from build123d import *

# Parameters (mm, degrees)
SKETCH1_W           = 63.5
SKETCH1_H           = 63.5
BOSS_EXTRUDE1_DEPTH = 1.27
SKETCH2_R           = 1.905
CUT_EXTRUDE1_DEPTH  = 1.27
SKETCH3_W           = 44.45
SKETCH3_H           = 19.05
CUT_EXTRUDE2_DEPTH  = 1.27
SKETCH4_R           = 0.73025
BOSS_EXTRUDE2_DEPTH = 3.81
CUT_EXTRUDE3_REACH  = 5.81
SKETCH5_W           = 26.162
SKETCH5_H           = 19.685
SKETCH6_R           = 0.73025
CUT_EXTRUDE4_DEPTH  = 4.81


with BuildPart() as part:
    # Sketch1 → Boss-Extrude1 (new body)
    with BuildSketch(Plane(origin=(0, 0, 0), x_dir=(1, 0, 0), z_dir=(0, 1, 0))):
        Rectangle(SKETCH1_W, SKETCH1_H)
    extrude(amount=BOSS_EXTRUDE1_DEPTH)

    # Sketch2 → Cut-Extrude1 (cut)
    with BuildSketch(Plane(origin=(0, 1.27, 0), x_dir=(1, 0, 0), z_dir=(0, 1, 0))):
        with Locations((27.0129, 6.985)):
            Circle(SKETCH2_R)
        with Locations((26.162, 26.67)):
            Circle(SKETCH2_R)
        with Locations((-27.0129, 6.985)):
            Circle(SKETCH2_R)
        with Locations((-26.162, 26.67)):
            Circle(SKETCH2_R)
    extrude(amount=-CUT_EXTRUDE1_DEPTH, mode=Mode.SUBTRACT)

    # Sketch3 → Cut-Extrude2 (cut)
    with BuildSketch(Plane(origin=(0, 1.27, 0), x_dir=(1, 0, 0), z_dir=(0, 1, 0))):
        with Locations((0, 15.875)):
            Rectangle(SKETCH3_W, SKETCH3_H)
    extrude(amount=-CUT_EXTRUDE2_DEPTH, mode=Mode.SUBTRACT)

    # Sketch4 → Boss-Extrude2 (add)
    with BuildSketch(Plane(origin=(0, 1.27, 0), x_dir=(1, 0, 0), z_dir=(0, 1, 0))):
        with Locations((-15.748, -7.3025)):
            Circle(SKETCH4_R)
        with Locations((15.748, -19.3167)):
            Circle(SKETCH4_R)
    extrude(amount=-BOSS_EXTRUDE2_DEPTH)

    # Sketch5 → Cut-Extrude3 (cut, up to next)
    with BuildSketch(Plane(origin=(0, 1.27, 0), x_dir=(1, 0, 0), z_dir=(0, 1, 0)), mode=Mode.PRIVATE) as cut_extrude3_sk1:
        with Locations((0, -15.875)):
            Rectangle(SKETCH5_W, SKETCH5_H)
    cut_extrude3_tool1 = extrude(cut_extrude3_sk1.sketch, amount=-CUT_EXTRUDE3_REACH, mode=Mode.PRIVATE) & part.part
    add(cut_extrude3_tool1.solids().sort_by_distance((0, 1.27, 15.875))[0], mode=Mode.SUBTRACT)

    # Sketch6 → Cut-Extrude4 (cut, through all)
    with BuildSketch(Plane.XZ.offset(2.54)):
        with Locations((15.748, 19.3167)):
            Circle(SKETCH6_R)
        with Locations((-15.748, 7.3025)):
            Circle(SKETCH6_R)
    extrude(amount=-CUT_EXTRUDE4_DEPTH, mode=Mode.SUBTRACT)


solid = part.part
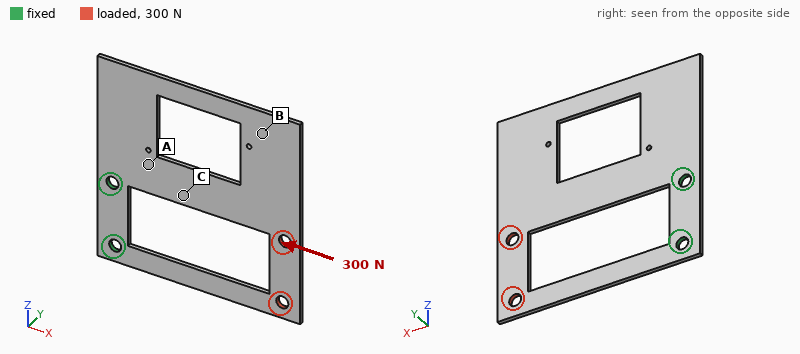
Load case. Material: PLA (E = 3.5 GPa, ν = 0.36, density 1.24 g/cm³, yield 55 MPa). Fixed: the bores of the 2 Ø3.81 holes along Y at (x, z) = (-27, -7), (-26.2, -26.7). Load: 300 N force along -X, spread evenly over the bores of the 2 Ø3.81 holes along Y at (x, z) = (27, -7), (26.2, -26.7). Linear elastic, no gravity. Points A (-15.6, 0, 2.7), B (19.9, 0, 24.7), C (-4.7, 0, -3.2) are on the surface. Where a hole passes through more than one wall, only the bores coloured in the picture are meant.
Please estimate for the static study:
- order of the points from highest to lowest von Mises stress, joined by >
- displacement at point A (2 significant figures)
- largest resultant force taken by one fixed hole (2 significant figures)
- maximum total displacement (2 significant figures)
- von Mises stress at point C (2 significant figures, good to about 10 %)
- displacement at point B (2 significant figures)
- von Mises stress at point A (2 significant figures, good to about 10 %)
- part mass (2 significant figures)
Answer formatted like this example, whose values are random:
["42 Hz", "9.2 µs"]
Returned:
["C > A > B", "0.084 mm", "150 N", "0.37 mm", "13 MPa", "0.074 mm", "6.4 MPa", "4.1 g"]
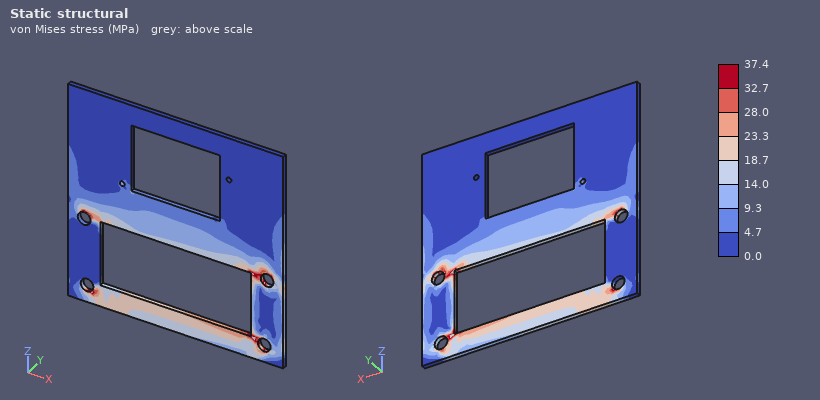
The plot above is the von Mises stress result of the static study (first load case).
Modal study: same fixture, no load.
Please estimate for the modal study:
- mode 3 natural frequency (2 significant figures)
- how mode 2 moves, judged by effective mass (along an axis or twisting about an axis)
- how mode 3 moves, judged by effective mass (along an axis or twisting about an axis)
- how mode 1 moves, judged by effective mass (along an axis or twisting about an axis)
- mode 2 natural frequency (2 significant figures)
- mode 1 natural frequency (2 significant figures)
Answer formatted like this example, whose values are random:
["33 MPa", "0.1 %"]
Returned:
["290 Hz", "twisting about X", "along Y", "along Y", "140 Hz", "65 Hz"]
